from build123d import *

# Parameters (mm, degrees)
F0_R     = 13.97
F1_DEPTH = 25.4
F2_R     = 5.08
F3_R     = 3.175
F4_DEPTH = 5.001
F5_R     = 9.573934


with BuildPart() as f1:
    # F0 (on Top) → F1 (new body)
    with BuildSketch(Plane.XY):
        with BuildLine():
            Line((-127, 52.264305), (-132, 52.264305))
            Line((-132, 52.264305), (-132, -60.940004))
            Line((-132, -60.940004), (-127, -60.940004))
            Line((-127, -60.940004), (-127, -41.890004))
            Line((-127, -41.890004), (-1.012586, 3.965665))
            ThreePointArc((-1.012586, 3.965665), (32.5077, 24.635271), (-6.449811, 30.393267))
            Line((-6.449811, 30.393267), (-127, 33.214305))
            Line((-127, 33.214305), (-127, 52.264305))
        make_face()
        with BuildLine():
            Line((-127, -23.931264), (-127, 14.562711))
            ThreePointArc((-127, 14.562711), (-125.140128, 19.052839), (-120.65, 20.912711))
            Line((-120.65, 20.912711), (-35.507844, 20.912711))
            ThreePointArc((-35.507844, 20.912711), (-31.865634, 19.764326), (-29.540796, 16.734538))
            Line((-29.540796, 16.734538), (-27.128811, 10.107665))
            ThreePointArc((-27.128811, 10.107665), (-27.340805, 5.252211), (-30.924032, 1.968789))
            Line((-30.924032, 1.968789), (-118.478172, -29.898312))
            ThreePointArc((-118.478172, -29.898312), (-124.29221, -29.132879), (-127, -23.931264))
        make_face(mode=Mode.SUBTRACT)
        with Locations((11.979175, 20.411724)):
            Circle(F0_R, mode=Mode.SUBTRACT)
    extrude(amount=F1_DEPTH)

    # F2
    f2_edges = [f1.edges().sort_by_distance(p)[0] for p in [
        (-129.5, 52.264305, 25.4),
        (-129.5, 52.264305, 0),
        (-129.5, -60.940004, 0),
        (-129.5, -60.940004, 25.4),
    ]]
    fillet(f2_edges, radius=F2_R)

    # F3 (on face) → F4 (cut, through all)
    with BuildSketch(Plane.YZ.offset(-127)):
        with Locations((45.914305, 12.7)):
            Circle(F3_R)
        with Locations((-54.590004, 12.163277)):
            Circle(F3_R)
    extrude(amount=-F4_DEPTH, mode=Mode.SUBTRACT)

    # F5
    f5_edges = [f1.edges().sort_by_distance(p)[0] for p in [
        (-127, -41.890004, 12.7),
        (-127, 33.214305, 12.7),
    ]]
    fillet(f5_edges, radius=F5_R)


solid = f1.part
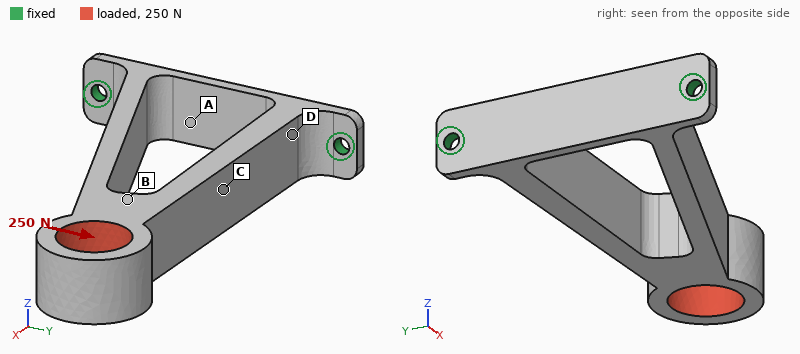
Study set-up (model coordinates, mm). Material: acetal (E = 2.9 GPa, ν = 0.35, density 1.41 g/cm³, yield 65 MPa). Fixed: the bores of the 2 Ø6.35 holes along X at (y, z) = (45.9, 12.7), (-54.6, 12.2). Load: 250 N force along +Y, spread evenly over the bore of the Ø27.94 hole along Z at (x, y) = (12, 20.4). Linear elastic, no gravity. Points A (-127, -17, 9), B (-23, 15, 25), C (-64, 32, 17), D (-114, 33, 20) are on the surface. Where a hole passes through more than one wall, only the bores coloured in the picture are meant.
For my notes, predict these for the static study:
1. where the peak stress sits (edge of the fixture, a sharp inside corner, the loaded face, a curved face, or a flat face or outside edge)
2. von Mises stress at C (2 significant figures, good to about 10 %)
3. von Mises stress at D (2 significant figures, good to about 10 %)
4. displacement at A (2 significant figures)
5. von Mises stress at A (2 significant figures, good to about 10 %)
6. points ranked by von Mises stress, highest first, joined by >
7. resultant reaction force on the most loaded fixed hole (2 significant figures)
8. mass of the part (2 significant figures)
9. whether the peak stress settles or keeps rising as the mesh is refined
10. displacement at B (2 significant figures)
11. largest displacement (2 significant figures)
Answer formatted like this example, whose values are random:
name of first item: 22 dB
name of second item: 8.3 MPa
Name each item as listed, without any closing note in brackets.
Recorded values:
where the peak stress sits: edge of the fixture
von Mises stress at C: 2.5 MPa
von Mises stress at D: 6.4 MPa
displacement at A: 0.21 mm
von Mises stress at A: 4.9 MPa
points ranked by von Mises stress, highest first, joined by >: D > A > C > B
resultant reaction force on the most loaded fixed hole: 440 N
mass of the part: 150 g
whether the peak stress settles or keeps rising as the mesh is refined: keeps rising
displacement at B: 0.72 mm
largest displacement: 1.3 mm
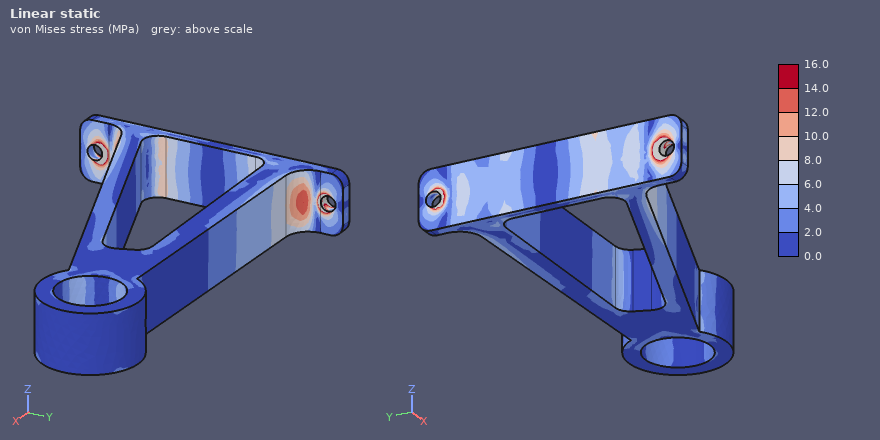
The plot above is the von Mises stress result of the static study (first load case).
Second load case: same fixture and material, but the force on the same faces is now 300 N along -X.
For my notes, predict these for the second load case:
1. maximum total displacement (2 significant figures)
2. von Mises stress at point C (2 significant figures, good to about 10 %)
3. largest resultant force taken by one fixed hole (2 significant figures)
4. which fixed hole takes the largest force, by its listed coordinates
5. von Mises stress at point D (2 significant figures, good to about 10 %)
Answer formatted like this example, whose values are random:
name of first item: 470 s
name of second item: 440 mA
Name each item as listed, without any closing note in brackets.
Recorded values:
maximum total displacement: 0.30 mm
von Mises stress at point C: 1.8 MPa
largest resultant force taken by one fixed hole: 240 N
which fixed hole takes the largest force, by its listed coordinates: (45.9, 12.7)
von Mises stress at point D: 3.8 MPa
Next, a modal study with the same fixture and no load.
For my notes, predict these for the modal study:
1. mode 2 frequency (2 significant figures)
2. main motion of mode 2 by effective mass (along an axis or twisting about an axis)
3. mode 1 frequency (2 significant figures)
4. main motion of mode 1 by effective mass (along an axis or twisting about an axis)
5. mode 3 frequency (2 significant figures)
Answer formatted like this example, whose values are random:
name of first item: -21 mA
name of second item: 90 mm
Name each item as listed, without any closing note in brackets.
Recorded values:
mode 2 frequency: 310 Hz
main motion of mode 2 by effective mass: along Y
mode 1 frequency: 76 Hz
main motion of mode 1 by effective mass: along Z
mode 3 frequency: 470 Hz
